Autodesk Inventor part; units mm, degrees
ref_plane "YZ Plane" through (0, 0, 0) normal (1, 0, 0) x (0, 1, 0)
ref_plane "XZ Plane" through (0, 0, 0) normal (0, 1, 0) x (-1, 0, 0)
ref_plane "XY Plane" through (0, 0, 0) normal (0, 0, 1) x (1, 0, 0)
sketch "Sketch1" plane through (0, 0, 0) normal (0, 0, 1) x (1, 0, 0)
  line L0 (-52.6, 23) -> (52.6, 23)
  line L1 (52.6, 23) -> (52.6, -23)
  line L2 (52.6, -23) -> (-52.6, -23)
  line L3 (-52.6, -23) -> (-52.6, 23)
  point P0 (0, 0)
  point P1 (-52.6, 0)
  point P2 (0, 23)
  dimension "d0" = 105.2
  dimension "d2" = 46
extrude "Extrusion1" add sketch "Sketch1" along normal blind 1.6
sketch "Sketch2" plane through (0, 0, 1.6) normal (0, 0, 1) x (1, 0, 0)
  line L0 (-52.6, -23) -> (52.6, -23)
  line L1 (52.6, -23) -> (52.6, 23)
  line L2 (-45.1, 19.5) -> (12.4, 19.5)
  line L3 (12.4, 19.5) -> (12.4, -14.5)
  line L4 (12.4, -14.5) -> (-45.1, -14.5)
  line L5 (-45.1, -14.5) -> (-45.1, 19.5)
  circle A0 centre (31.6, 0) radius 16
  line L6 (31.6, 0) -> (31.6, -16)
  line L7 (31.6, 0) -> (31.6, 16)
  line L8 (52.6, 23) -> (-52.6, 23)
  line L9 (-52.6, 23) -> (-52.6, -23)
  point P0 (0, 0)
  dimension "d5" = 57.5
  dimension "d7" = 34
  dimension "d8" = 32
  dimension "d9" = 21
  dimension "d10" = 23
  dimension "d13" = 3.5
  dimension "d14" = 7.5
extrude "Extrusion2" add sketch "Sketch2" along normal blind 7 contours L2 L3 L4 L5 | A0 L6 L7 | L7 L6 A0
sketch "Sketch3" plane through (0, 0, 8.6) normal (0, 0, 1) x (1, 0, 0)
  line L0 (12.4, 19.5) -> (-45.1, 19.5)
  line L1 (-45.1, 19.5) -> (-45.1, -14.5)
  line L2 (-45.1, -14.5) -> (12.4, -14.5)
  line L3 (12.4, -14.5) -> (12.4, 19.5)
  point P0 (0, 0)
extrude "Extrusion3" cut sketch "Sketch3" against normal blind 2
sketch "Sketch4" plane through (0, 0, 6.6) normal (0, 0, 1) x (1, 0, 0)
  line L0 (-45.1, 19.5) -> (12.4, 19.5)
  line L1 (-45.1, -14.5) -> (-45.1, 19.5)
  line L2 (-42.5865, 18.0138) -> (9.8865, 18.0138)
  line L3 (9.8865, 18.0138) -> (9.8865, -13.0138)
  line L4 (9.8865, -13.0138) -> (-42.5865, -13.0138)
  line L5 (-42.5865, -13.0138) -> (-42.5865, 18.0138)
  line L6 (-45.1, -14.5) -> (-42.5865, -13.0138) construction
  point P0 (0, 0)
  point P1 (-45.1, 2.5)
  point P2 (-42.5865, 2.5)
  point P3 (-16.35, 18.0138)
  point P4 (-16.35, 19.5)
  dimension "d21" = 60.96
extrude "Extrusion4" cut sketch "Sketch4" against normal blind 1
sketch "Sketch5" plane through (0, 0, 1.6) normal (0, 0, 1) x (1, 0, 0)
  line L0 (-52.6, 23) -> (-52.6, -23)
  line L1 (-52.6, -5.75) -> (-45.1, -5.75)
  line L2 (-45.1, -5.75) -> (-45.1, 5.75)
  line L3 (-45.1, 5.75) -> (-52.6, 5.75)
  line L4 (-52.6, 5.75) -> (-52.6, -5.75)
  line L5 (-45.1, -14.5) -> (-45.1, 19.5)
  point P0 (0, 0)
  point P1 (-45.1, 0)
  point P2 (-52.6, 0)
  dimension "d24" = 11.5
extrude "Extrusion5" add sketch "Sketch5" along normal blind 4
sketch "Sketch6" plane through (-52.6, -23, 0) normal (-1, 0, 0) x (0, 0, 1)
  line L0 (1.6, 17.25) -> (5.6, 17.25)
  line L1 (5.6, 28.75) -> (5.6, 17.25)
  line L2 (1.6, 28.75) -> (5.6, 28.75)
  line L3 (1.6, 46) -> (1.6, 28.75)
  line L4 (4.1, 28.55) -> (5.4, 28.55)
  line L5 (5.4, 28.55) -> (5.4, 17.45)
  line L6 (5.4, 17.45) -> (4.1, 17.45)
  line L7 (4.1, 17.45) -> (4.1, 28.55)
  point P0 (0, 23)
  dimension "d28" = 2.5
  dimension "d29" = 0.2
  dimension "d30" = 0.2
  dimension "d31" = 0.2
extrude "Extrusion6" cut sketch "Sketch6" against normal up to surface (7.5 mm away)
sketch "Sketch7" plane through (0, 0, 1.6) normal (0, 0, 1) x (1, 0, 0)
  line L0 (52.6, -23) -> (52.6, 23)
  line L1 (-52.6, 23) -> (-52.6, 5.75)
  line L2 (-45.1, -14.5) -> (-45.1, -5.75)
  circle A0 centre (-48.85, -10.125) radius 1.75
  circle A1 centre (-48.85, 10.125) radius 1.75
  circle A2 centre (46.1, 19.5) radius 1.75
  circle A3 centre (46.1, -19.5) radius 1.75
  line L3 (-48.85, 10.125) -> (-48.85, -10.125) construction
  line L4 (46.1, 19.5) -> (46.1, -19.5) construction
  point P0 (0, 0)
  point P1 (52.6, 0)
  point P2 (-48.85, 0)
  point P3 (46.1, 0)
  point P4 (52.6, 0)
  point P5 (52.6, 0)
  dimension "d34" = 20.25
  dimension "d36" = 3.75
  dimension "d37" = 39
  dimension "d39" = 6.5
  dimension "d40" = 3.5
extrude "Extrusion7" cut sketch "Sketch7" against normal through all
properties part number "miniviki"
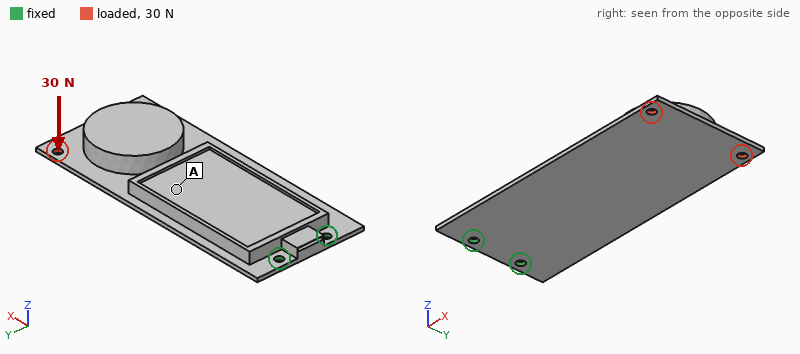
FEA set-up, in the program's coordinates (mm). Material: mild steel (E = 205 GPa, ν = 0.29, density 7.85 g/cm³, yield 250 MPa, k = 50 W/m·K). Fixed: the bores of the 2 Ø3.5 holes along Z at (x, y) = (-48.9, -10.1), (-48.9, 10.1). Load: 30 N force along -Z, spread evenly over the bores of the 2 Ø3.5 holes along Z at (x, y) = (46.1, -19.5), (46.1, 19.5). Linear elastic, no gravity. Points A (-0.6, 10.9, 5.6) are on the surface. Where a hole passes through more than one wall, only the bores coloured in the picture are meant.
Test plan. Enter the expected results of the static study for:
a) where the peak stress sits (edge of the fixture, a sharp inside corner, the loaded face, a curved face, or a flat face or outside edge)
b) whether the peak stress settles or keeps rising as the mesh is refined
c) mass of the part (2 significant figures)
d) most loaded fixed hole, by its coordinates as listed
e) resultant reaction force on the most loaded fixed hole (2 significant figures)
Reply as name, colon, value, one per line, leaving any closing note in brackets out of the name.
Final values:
where the peak stress sits: edge of the fixture
whether the peak stress settles or keeps rising as the mesh is refined: keeps rising
mass of the part: 170 g
most loaded fixed hole, by its coordinates as listed: (-48.9, 10.1)
resultant reaction force on the most loaded fixed hole: 32 N
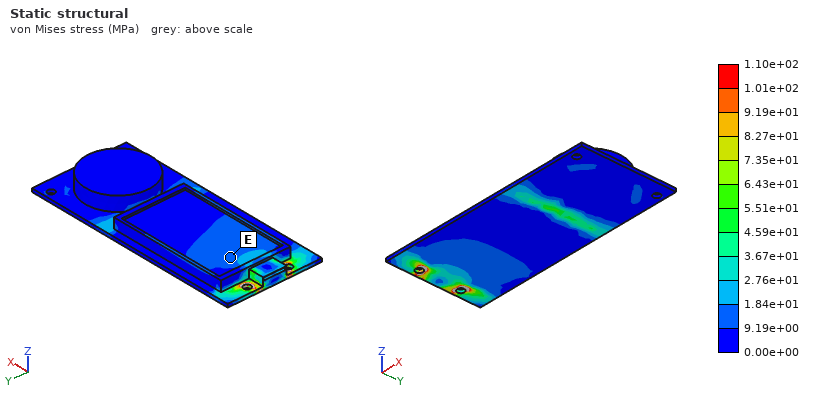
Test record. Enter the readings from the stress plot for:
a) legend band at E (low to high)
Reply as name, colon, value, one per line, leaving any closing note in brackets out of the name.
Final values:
legend band at E: 9.19e+00 to 1.84e+01 MPa
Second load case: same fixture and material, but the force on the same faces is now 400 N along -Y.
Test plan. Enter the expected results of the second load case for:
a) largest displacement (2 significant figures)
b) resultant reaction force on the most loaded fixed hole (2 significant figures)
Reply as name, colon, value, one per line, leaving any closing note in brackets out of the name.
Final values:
largest displacement: 74 µm
resultant reaction force on the most loaded fixed hole: 1.7 kN
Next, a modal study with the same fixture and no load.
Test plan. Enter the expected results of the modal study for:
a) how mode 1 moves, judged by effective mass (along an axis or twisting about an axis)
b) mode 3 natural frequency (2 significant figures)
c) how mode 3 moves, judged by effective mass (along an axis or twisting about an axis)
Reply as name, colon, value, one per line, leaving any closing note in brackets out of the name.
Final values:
how mode 1 moves, judged by effective mass: along Z
mode 3 natural frequency: 1700 Hz
how mode 3 moves, judged by effective mass: along Y
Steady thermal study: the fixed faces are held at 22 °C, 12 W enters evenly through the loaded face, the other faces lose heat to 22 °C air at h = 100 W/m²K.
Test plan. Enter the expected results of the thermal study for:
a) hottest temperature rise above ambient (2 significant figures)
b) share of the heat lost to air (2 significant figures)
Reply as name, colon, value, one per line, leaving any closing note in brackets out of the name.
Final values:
hottest temperature rise above ambient: 68 K
share of the heat lost to air: 96 %
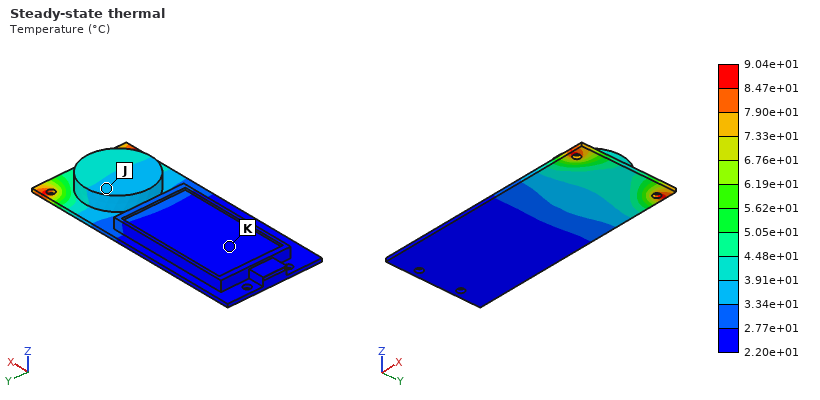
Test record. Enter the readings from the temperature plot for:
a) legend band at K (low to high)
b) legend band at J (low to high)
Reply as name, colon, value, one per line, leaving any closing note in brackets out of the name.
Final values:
legend band at K: 2.20e+01 to 2.77e+01 °C
legend band at J: 3.34e+01 to 3.91e+01 °C
